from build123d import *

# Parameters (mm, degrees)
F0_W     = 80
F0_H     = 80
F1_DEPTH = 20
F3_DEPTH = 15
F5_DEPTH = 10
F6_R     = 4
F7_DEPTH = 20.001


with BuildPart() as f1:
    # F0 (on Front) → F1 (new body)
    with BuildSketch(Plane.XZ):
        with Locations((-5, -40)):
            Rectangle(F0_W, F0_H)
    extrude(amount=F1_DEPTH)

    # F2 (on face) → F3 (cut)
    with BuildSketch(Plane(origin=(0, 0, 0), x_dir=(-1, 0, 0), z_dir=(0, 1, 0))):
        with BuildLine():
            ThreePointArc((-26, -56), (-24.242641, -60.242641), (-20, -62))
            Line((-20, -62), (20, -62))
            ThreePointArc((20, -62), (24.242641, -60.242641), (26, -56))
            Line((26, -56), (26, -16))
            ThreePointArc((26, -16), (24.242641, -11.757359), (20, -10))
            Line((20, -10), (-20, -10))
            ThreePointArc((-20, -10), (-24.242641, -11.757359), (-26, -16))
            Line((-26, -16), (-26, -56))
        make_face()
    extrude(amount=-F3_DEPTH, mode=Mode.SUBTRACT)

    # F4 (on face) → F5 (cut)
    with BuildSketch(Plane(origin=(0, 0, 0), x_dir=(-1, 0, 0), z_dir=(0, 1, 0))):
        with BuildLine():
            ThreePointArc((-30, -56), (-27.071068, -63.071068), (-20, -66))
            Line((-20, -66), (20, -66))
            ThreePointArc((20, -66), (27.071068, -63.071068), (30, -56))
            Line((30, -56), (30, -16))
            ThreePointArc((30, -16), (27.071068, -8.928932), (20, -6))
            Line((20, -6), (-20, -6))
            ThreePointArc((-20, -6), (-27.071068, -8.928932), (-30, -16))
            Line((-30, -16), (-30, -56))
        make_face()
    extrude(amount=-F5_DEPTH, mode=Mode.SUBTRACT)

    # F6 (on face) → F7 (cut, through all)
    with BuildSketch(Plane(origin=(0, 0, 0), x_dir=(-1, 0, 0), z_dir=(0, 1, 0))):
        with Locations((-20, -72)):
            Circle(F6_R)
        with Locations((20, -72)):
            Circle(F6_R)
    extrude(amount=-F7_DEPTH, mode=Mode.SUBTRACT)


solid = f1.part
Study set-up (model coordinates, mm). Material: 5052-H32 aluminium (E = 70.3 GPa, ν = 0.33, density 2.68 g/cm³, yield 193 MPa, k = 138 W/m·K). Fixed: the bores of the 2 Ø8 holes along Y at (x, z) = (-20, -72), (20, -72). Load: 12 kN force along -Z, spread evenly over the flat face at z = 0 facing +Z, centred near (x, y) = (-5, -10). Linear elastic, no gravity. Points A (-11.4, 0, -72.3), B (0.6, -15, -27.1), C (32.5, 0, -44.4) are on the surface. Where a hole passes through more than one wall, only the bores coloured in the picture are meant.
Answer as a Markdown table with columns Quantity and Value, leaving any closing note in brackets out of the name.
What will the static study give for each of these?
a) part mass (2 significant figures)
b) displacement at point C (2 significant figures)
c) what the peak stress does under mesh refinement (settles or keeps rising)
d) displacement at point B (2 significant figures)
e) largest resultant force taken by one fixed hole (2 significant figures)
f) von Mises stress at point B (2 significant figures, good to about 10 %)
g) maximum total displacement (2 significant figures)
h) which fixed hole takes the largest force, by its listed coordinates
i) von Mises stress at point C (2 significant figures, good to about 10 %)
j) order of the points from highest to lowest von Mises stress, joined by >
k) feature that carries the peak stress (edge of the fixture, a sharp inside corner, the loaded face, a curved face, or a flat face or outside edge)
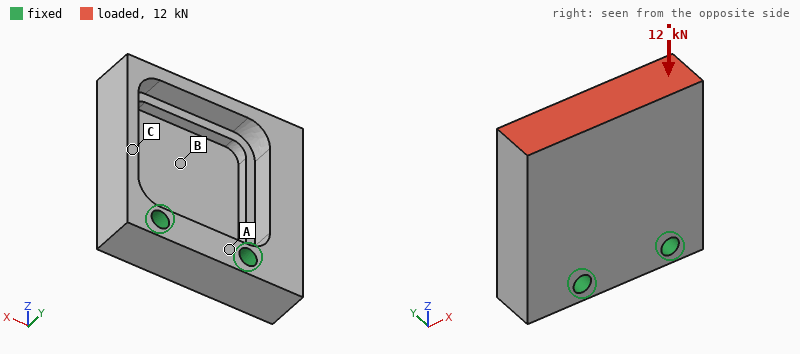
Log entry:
| Quantity | Value |
|---|---|
| part mass | 210 g |
| displacement at point C | 0.033 mm |
| what the peak stress does under mesh refinement | keeps rising |
| displacement at point B | 0.039 mm |
| largest resultant force taken by one fixed hole | 7.1 kN |
| von Mises stress at point B | 37 MPa |
| maximum total displacement | 0.19 mm |
| which fixed hole takes the largest force, by its listed coordinates | (-20, -72) |
| von Mises stress at point C | 62 MPa |
| order of the points from highest to lowest von Mises stress, joined by > | C > B > A |
| feature that carries the peak stress | edge of the fixture |
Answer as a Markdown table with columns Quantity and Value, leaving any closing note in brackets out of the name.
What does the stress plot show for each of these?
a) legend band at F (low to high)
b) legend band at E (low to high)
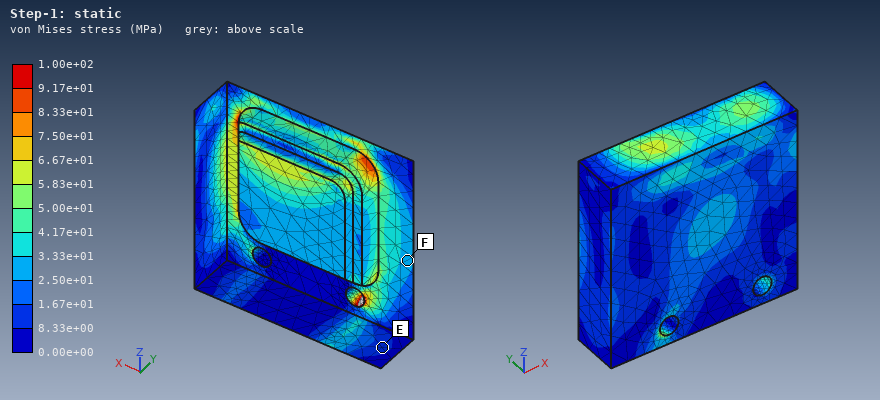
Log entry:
| Quantity | Value |
|---|---|
| legend band at F | 2.50e+01 to 3.33e+01 MPa |
| legend band at E | 8.33e+00 to 1.67e+01 MPa |
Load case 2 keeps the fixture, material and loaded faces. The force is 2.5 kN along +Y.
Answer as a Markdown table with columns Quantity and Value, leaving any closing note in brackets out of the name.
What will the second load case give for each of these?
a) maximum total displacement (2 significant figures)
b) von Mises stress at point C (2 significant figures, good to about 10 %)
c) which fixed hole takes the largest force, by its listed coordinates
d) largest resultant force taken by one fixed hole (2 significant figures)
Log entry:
| Quantity | Value |
|---|---|
| maximum total displacement | 0.33 mm |
| von Mises stress at point C | 94 MPa |
| which fixed hole takes the largest force, by its listed coordinates | (-20, -72) |
| largest resultant force taken by one fixed hole | 1.6 kN |
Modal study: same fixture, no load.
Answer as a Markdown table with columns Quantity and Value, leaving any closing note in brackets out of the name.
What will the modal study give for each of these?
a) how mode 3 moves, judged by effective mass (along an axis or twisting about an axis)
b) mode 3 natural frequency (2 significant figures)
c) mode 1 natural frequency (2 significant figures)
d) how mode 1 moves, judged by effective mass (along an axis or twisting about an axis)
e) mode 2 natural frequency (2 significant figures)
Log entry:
| Quantity | Value |
|---|---|
| how mode 3 moves, judged by effective mass | along X |
| mode 3 natural frequency | 5200 Hz |
| mode 1 natural frequency | 2000 Hz |
| how mode 1 moves, judged by effective mass | along Y |
| mode 2 natural frequency | 3000 Hz |
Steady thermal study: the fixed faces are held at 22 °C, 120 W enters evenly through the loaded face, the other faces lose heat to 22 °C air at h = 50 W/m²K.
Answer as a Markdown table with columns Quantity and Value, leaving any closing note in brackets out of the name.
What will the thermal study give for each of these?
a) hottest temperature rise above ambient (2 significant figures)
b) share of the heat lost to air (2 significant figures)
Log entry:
| Quantity | Value |
|---|---|
| hottest temperature rise above ambient | 77 K |
| share of the heat lost to air | 25 % |
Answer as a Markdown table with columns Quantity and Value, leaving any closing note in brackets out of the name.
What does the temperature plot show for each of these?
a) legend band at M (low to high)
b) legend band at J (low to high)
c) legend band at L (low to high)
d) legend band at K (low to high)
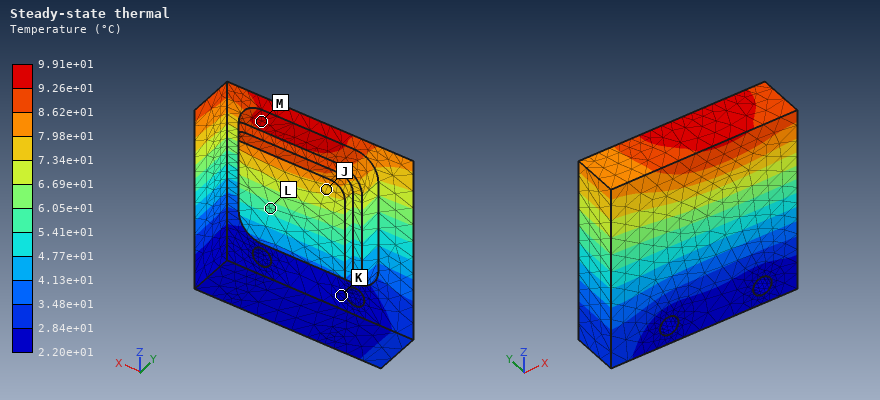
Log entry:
| Quantity | Value |
|---|---|
| legend band at M | 9.26e+01 to 9.91e+01 °C |
| legend band at J | 7.34e+01 to 7.98e+01 °C |
| legend band at L | 5.41e+01 to 6.05e+01 °C |
| legend band at K | 2.20e+01 to 2.84e+01 °C |
